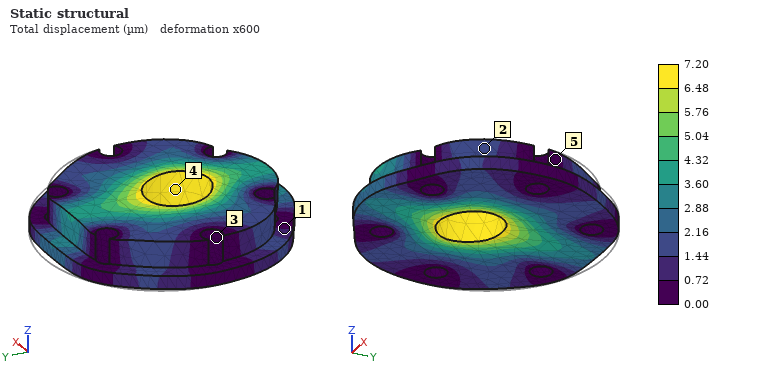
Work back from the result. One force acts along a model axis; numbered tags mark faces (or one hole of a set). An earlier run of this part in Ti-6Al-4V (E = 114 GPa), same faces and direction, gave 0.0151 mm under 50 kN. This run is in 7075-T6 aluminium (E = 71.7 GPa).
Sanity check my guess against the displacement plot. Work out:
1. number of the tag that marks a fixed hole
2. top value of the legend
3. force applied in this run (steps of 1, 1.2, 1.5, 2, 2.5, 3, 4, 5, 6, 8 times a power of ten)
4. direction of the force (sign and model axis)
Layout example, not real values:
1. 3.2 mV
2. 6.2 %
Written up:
1. 3
2. 7.20 µm
3. 15 kN
4. -Y
